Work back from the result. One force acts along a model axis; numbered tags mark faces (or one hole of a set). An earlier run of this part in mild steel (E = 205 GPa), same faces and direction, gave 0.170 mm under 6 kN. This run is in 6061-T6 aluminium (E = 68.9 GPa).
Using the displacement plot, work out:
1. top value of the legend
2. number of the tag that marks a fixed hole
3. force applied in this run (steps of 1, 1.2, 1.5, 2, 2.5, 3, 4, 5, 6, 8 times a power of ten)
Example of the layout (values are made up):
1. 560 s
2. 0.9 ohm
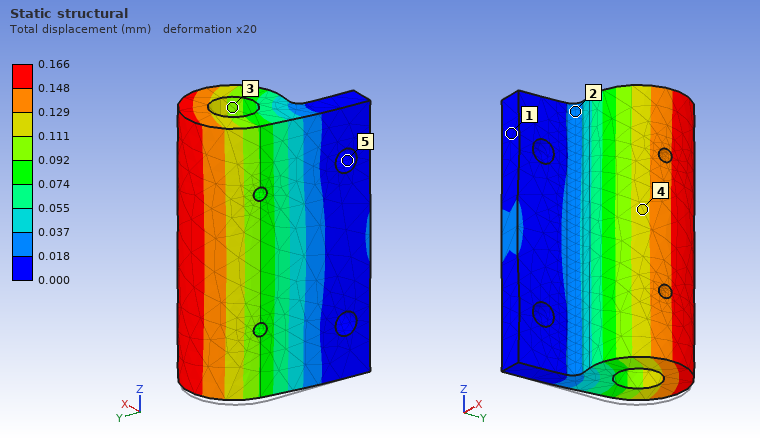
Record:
1. 0.166 mm
2. 5
3. 2 kN
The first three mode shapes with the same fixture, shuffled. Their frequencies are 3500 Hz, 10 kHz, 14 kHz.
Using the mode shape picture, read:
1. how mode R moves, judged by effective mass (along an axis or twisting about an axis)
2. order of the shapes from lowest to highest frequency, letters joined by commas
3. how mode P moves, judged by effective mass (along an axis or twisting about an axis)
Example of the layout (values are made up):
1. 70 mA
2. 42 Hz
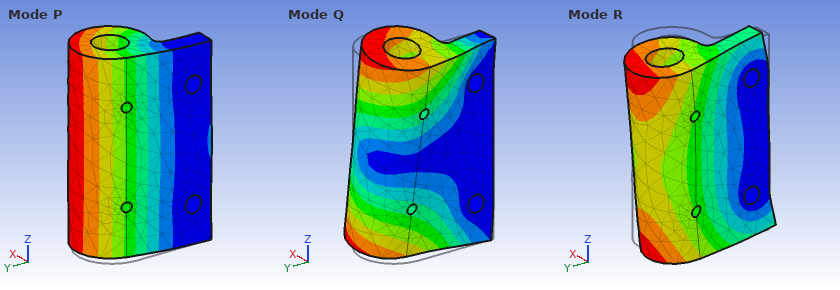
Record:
1. along Z
2. P, Q, R
3. along X
